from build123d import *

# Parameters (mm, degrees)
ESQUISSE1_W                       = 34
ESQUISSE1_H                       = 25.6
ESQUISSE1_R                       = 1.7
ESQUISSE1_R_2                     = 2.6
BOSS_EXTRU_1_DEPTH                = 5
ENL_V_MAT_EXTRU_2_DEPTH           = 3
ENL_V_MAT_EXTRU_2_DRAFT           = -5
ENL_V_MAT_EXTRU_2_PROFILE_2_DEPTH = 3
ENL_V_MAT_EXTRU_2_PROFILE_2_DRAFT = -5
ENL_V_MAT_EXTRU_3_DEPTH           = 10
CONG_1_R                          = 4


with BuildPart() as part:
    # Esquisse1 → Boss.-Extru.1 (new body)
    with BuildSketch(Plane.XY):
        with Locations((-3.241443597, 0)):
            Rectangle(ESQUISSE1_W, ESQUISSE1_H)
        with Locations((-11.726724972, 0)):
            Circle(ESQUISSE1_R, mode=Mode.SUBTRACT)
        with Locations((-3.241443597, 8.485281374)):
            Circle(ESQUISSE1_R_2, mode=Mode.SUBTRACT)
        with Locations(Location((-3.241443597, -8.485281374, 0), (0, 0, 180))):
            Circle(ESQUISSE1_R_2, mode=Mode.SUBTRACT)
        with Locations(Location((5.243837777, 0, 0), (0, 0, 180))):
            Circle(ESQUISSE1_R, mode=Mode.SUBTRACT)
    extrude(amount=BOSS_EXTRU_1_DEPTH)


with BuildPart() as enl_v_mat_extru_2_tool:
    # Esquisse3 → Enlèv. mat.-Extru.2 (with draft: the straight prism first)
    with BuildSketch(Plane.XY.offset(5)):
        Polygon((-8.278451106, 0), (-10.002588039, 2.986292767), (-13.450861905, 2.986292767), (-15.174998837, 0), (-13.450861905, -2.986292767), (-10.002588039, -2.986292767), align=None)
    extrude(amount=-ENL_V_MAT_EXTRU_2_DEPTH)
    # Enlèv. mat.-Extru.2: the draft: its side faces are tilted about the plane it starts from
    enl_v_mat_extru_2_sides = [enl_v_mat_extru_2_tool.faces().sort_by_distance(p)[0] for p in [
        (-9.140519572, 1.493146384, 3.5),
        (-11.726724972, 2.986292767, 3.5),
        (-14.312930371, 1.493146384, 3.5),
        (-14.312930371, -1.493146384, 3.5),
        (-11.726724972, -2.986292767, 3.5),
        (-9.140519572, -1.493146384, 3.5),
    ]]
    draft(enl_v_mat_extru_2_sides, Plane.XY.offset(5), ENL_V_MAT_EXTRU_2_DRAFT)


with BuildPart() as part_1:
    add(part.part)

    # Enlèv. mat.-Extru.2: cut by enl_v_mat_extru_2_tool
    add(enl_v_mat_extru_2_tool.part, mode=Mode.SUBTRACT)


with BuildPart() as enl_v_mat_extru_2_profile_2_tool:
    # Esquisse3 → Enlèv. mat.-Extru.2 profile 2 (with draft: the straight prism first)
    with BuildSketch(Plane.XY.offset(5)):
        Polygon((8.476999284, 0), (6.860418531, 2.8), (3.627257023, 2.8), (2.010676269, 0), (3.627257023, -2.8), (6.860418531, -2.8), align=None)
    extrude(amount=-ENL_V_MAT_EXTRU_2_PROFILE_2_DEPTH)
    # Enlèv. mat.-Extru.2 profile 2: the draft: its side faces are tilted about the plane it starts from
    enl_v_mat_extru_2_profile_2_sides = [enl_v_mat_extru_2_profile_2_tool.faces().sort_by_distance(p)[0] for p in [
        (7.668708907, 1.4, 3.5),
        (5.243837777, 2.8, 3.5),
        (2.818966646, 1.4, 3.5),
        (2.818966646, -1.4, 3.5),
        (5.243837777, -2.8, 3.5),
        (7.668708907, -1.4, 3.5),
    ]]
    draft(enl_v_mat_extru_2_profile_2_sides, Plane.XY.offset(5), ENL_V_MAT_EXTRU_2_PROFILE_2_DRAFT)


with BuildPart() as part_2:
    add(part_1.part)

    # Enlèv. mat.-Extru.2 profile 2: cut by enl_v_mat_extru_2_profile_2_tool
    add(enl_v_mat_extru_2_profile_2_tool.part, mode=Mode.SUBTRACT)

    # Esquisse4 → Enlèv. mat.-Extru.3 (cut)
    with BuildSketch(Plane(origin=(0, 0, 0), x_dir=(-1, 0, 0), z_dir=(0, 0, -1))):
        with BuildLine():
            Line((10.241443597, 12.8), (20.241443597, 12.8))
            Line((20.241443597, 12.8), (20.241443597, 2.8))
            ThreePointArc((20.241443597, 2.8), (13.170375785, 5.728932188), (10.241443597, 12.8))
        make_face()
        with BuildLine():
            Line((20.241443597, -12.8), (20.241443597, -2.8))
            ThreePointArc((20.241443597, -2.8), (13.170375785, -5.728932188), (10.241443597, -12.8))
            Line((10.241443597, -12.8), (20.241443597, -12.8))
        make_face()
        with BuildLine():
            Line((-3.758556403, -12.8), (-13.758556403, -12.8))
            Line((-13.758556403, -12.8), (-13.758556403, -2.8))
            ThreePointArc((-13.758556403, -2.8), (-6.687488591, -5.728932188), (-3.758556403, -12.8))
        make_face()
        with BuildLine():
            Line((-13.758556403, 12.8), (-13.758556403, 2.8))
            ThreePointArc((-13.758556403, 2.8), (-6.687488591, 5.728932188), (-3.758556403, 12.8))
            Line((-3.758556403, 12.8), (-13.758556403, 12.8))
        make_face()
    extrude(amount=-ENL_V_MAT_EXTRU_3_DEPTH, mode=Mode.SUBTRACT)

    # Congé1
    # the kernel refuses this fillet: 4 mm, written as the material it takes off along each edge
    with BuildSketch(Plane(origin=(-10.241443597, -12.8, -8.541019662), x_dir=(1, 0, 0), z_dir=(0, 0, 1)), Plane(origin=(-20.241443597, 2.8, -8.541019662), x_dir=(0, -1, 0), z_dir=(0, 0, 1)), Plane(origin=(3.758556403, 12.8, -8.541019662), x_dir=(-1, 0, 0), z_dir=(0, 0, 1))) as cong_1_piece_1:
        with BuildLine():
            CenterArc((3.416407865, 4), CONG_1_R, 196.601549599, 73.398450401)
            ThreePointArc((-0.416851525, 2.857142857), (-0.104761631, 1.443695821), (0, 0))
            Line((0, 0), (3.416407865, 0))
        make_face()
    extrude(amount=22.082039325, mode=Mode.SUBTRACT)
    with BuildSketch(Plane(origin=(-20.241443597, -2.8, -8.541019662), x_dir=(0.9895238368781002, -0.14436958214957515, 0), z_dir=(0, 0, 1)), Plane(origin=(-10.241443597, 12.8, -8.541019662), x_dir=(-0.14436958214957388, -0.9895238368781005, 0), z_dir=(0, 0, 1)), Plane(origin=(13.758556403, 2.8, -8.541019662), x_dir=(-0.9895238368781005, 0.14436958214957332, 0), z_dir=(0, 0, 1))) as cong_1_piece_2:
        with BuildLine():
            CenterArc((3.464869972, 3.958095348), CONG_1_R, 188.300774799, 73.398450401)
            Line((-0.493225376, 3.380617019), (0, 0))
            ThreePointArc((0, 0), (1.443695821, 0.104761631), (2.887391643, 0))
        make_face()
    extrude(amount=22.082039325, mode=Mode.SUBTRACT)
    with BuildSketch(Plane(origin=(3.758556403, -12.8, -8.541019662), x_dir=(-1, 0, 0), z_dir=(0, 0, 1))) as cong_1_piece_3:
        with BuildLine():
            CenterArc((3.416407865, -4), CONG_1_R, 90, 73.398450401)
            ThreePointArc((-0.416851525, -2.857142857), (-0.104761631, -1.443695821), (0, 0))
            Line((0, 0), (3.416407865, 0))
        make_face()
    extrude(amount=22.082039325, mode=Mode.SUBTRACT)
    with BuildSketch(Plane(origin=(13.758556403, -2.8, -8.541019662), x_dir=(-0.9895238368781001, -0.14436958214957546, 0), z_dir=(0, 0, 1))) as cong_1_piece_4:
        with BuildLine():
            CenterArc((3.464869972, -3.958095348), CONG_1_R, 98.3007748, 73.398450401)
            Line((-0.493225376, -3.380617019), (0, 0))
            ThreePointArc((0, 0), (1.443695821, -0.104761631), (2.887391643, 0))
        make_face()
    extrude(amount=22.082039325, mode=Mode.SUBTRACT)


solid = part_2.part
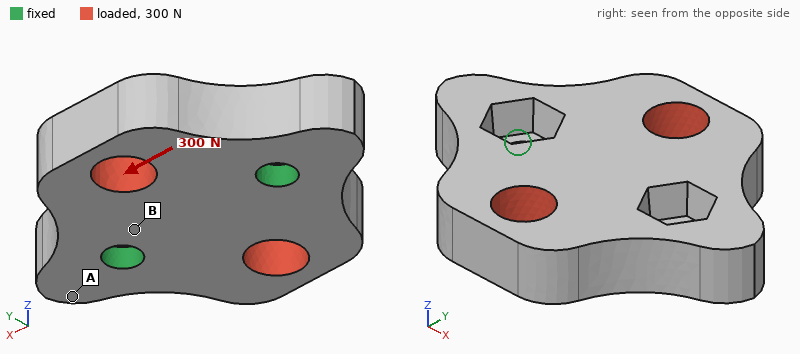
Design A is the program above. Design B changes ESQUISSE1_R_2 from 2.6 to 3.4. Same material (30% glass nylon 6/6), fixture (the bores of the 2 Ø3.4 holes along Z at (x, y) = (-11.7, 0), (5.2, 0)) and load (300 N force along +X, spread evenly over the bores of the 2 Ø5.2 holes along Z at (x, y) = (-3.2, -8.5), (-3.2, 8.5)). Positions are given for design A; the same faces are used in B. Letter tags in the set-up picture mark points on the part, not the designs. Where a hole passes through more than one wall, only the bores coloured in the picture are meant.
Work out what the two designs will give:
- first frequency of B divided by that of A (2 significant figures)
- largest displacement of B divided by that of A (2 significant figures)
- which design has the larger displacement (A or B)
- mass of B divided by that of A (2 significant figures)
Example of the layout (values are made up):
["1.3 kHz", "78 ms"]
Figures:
["1.1", "1.4", "B", "0.93"]
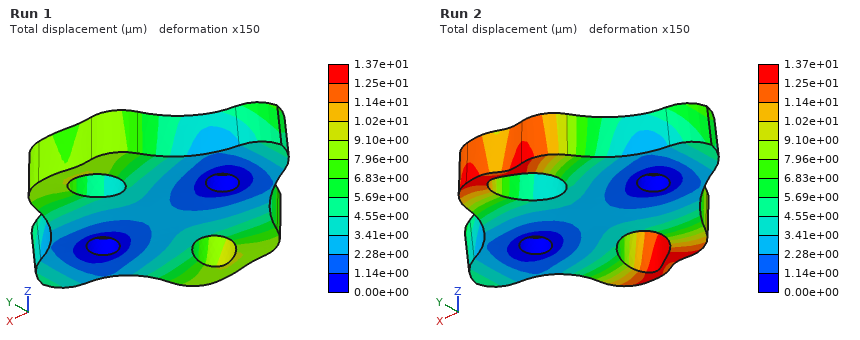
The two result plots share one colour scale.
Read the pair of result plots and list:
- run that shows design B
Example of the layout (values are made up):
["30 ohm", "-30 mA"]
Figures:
["Run 2"]
